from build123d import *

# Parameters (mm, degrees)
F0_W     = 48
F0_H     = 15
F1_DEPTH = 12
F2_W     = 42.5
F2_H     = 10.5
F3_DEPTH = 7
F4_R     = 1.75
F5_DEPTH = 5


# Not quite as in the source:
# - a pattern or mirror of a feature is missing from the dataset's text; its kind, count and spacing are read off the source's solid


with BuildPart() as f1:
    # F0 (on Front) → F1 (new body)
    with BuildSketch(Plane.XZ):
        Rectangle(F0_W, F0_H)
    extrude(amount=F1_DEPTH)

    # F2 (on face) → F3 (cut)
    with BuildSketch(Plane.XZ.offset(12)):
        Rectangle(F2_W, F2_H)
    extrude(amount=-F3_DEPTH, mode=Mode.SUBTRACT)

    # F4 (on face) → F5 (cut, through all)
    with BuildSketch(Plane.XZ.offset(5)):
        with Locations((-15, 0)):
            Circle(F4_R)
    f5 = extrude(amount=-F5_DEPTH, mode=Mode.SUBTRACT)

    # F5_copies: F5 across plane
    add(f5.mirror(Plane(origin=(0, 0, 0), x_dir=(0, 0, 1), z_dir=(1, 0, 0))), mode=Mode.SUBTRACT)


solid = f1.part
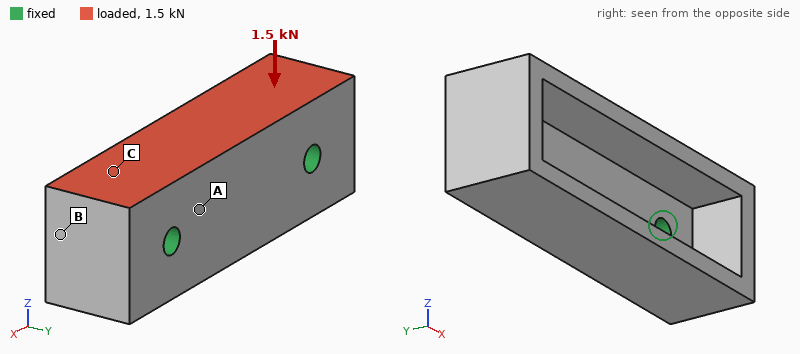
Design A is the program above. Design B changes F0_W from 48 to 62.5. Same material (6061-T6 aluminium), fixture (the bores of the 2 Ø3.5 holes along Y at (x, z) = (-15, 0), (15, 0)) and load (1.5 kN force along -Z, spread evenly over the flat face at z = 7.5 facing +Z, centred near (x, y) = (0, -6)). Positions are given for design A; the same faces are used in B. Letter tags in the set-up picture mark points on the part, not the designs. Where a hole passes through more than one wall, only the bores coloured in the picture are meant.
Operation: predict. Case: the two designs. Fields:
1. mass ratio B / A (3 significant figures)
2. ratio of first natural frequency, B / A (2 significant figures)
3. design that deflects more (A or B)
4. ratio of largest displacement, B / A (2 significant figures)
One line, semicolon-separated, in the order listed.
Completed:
1.48; 0.76; A; 0.75
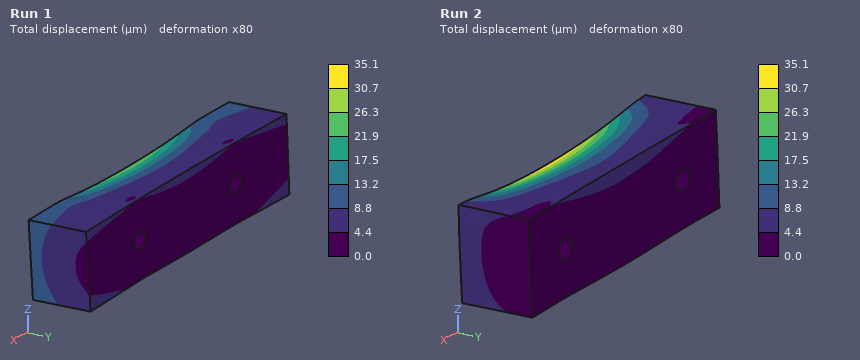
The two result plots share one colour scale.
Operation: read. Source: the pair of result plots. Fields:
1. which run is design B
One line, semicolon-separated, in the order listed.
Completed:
Run 1
